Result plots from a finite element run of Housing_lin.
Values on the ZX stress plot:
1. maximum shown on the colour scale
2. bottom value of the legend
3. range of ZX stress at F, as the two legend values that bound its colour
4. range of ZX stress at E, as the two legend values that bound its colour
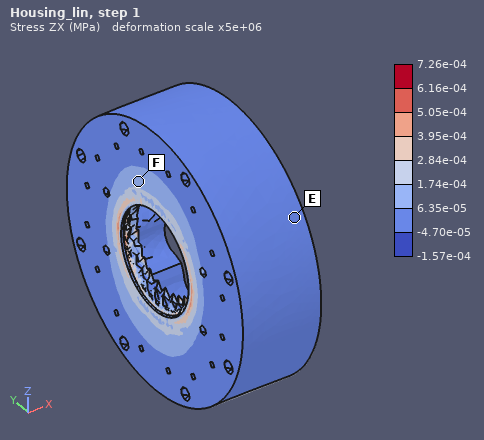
7.26e-04 MPa
-1.57e-04 MPa
6.35e-05 to 1.74e-04 MPa
-4.70e-05 to 6.35e-05 MPa
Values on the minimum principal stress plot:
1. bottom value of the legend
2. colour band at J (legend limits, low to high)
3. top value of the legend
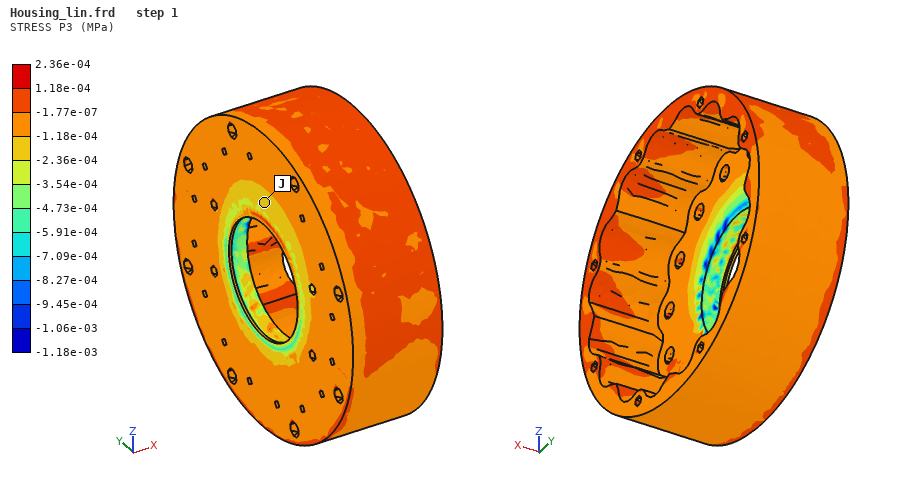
-1.18e-03 MPa
-2.36e-04 to -1.18e-04 MPa
2.36e-04 MPa
